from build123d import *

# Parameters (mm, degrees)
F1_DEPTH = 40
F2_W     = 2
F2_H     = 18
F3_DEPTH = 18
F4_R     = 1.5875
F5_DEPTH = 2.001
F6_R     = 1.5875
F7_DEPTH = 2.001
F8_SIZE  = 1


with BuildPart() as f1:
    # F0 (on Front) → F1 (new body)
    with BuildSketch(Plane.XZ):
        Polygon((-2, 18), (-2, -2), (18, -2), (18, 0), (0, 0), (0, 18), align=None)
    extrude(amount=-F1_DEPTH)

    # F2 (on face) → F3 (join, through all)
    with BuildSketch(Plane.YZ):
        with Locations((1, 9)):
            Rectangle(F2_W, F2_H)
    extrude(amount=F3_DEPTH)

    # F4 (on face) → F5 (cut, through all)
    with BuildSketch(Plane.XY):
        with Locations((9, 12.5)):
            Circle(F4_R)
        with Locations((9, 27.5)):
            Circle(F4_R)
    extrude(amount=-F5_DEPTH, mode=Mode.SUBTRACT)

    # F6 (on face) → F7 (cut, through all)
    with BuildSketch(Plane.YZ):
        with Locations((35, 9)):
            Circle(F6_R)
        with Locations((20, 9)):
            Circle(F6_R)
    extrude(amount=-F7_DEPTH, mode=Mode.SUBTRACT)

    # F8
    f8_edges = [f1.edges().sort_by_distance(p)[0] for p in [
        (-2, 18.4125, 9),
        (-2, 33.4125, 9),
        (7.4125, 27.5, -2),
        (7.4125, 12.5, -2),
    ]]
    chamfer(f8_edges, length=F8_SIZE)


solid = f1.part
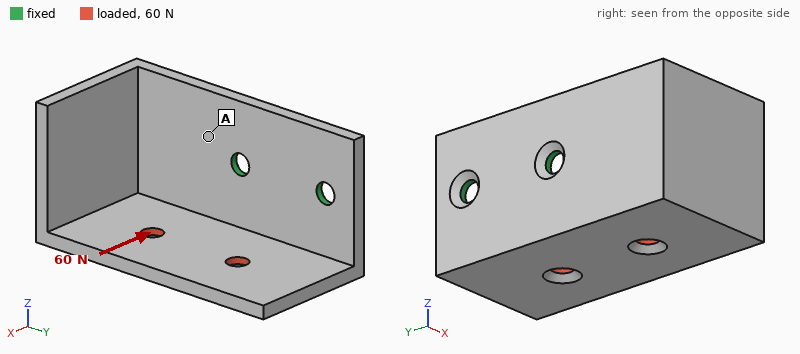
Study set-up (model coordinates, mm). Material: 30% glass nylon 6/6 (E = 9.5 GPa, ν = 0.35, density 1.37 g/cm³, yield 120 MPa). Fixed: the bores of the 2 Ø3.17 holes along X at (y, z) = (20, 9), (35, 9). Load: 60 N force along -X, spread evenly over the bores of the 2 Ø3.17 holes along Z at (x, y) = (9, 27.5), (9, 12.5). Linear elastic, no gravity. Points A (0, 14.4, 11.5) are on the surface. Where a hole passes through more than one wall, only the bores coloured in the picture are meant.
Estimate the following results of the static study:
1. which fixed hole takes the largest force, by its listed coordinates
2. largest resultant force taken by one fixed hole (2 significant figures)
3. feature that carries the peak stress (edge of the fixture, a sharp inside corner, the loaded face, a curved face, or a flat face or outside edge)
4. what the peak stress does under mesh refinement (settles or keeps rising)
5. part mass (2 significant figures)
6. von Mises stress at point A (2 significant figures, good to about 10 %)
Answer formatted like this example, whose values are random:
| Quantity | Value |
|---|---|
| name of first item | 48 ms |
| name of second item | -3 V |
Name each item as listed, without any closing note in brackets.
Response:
| Quantity | Value |
|---|---|
| which fixed hole takes the largest force, by its listed coordinates | (20, 9) |
| largest resultant force taken by one fixed hole | 54 N |
| feature that carries the peak stress | edge of the fixture |
| what the peak stress does under mesh refinement | keeps rising |
| part mass | 4.9 g |
| von Mises stress at point A | 12 MPa |
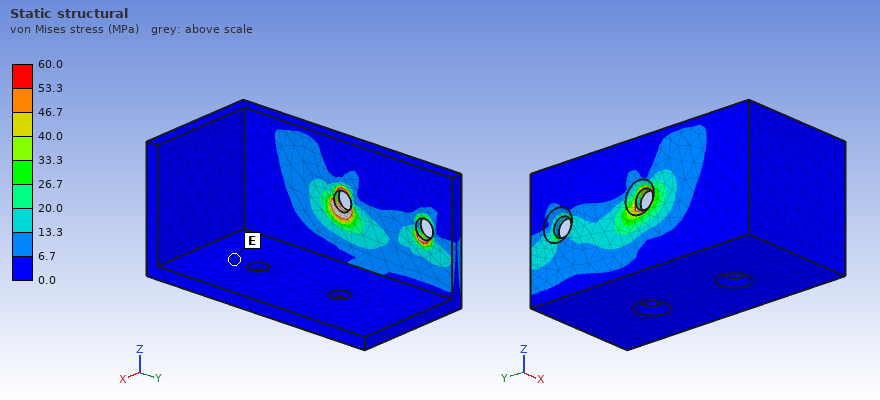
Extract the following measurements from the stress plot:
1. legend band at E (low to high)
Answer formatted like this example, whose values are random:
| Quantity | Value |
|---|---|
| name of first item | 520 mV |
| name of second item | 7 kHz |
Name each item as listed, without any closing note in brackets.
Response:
| Quantity | Value |
|---|---|
| legend band at E | 0.0 to 6.7 MPa |
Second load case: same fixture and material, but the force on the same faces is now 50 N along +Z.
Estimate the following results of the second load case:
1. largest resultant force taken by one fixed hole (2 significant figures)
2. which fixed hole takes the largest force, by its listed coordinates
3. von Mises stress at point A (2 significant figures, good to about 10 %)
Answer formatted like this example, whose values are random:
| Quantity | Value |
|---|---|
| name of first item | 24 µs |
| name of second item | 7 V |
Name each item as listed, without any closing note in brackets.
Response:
| Quantity | Value |
|---|---|
| largest resultant force taken by one fixed hole | 50 N |
| which fixed hole takes the largest force, by its listed coordinates | (20, 9) |
| von Mises stress at point A | 13 MPa |
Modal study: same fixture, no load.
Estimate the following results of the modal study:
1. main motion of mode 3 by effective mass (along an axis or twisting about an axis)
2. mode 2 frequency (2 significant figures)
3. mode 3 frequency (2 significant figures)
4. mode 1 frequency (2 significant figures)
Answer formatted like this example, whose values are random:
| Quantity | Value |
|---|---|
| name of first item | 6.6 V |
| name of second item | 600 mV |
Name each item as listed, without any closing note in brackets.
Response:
| Quantity | Value |
|---|---|
| main motion of mode 3 by effective mass | along X |
| mode 2 frequency | 1300 Hz |
| mode 3 frequency | 2100 Hz |
| mode 1 frequency | 980 Hz |
